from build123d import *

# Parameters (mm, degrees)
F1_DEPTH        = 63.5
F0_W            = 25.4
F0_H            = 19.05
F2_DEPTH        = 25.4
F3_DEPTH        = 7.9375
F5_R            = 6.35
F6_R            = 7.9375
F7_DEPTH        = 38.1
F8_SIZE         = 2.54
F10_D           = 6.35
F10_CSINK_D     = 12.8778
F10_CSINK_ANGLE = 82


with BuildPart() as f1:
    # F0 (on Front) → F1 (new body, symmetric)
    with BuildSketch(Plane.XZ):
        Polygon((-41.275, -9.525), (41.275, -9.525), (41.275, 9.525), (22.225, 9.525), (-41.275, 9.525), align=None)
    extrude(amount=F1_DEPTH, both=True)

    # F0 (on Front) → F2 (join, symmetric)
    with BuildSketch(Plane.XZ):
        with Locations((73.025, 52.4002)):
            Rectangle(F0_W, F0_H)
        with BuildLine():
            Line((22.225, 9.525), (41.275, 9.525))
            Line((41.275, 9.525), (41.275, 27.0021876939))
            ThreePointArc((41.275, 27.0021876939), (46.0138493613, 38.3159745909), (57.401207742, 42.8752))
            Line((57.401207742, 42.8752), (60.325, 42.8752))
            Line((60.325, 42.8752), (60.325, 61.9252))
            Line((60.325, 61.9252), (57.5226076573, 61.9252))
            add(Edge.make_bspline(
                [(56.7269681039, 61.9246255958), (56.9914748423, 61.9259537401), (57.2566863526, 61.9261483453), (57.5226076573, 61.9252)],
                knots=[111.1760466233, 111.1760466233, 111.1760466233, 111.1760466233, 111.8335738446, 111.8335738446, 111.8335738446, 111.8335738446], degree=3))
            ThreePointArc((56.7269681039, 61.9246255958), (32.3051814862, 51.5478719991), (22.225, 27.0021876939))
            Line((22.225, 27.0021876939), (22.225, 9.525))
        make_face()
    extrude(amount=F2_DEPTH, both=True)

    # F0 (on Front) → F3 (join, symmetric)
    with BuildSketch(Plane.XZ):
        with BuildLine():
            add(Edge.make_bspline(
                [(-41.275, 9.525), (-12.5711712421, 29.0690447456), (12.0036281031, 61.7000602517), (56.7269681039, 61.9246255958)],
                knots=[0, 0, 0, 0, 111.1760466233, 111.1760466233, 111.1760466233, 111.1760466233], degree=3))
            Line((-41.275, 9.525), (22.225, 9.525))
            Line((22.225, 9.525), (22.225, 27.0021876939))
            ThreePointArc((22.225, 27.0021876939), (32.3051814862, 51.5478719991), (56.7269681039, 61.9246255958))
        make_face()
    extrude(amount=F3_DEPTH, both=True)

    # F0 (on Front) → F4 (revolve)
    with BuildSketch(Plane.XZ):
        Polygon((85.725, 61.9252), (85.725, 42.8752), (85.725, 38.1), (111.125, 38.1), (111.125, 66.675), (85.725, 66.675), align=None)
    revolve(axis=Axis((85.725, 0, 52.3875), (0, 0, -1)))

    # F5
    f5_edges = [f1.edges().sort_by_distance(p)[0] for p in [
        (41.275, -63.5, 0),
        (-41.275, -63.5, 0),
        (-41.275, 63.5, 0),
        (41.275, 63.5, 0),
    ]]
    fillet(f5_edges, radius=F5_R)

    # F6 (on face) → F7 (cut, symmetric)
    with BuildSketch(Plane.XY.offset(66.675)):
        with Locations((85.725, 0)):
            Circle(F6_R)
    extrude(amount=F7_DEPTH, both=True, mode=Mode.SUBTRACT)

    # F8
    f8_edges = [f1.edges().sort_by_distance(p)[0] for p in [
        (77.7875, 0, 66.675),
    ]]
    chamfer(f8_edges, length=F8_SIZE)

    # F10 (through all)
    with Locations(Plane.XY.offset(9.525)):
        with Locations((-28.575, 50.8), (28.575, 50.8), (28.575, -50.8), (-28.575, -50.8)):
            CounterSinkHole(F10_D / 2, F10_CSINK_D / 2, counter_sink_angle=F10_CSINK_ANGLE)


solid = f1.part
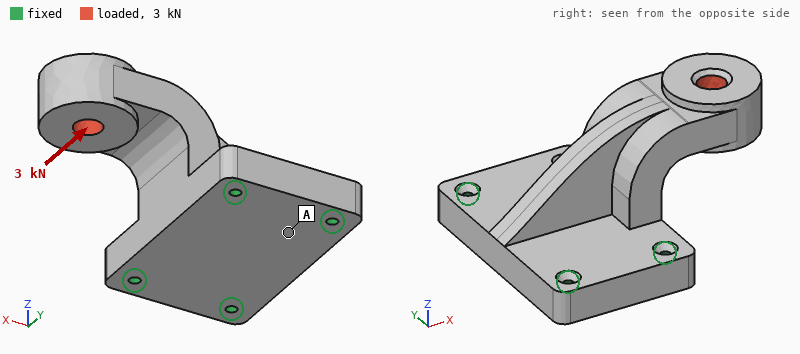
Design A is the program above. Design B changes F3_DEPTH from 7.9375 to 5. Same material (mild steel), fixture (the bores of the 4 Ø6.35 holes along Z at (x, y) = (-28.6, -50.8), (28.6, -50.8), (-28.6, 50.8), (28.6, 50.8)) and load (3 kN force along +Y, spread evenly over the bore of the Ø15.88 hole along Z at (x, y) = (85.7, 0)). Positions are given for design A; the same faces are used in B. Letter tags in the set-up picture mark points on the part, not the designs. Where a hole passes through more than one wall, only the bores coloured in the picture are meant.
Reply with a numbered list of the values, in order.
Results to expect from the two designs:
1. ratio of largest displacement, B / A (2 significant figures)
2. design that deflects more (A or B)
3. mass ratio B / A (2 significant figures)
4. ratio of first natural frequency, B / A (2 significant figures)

1. 1.1
2. B
3. 0.97
4. 0.95
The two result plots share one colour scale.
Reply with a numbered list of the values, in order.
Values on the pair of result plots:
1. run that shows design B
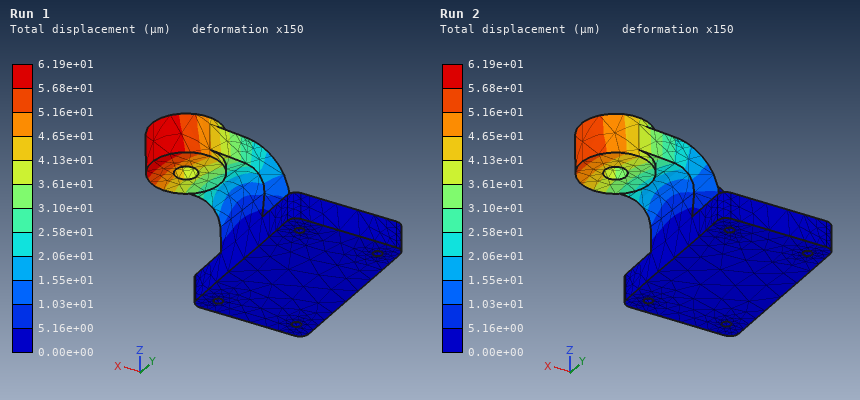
1. Run 1
